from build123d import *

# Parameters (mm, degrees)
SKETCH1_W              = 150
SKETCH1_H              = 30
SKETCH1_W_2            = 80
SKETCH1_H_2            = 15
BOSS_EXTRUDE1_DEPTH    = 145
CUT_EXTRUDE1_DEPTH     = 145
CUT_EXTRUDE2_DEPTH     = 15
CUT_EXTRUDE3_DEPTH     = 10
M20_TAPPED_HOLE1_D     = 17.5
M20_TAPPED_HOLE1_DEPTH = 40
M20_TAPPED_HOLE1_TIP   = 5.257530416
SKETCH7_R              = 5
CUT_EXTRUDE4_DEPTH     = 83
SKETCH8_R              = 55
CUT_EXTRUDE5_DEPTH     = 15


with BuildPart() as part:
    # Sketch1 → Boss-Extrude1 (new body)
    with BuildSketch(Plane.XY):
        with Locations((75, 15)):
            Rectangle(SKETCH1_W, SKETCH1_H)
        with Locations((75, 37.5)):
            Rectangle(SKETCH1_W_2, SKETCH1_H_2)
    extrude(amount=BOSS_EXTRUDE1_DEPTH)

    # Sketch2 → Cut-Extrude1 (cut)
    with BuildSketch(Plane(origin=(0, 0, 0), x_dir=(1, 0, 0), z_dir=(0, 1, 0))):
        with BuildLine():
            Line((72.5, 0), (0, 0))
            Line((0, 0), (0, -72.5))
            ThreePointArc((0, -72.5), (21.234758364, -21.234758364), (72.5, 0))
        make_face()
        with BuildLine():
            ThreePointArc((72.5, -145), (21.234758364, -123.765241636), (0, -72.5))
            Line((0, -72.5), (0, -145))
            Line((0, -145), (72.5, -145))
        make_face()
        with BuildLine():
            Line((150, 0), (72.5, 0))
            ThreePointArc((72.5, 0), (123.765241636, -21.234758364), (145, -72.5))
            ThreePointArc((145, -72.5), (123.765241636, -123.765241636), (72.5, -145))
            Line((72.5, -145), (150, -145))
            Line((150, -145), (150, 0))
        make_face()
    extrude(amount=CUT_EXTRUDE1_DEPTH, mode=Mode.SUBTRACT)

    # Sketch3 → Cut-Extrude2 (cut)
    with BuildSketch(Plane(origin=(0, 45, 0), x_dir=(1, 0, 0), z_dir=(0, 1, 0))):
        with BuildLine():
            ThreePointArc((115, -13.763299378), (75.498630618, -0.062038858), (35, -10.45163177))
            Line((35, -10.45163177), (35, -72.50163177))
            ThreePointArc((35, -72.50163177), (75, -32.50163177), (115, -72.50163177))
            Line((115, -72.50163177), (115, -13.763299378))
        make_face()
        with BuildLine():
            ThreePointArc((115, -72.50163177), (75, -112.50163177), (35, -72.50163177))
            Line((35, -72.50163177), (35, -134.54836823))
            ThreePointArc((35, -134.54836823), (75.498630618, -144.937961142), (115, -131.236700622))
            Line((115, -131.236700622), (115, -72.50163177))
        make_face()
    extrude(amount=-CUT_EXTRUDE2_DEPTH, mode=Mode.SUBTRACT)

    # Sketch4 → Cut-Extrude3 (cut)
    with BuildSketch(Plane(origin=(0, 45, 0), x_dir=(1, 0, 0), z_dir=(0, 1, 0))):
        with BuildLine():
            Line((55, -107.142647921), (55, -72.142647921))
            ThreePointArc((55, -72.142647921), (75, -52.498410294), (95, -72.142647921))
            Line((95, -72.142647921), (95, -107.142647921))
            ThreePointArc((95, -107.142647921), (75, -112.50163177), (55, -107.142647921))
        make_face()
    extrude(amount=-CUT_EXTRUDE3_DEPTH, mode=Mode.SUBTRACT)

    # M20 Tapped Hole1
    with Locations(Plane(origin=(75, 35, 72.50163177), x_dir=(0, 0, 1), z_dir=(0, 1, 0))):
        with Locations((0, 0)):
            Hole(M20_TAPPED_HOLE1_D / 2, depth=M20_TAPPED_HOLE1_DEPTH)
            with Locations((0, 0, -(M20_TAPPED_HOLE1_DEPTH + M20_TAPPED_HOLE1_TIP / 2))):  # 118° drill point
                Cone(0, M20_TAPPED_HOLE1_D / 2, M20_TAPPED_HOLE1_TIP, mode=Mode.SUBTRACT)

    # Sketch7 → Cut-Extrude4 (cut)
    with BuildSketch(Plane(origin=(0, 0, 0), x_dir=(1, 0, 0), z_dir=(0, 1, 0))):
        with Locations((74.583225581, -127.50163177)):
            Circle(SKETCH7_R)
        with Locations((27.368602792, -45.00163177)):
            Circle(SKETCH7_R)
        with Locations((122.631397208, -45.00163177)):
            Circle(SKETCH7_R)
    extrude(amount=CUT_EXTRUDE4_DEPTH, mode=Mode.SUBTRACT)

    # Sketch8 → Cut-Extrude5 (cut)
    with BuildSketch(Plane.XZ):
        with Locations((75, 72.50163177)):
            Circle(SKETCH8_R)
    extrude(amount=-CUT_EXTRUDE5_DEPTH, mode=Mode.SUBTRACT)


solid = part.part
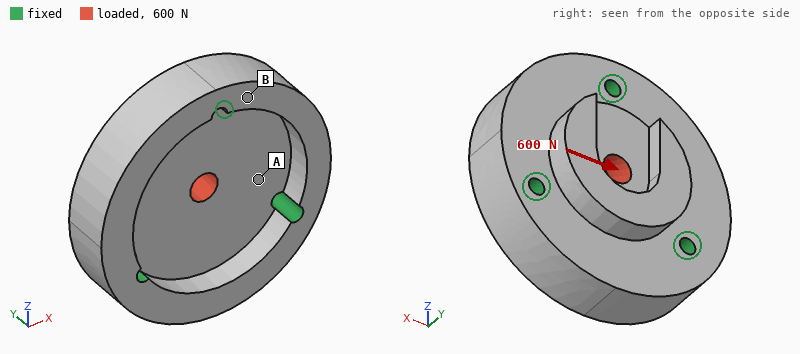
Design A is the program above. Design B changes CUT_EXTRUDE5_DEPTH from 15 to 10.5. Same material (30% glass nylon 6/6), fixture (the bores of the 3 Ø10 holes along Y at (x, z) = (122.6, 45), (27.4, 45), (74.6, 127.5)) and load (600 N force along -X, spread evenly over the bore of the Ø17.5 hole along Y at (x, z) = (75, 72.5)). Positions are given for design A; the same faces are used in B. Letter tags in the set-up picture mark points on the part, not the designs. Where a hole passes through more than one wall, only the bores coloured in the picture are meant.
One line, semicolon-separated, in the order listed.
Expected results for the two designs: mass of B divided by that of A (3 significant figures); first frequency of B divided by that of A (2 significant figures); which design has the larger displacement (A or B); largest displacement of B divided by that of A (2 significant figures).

1.10; 1.0; A; 0.81
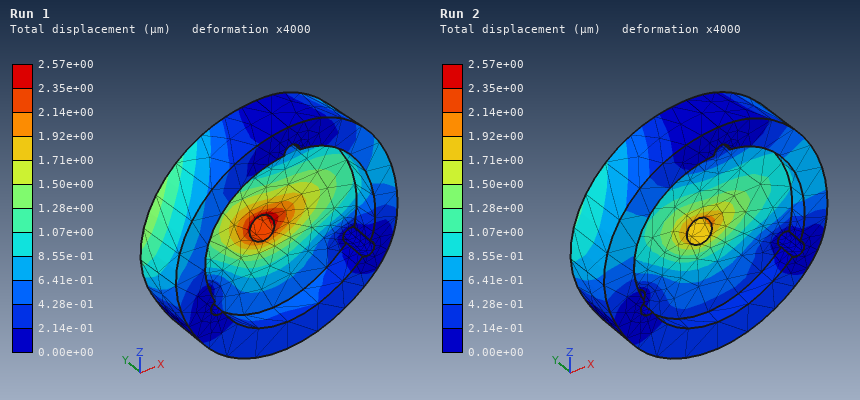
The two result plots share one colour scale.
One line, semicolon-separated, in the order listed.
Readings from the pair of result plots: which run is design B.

Run 2
